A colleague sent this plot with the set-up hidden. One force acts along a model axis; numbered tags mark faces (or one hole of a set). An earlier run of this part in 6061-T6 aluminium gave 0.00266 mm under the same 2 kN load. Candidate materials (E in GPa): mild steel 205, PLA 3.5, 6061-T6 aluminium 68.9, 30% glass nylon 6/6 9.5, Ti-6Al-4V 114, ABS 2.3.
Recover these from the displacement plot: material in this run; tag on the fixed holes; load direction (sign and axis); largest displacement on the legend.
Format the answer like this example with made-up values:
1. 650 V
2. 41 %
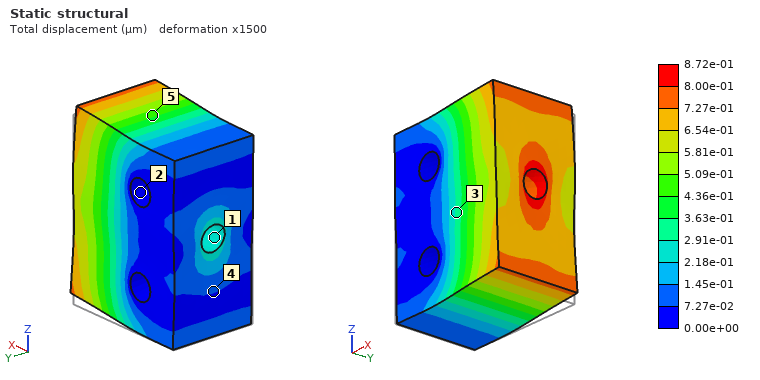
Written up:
1. mild steel
2. 2
3. +Z
4. 8.72e-01 µm
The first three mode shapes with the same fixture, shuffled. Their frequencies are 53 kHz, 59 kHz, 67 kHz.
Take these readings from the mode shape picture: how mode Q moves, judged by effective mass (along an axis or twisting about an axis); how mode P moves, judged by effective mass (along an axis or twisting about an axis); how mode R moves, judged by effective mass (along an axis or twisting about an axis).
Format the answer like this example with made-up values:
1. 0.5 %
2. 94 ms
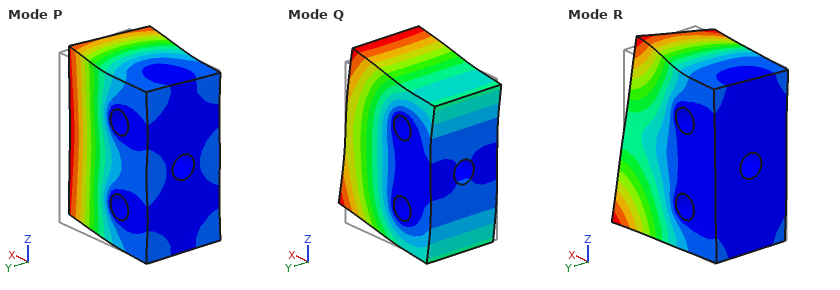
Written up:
1. along Z
2. along Y
3. twisting about X
